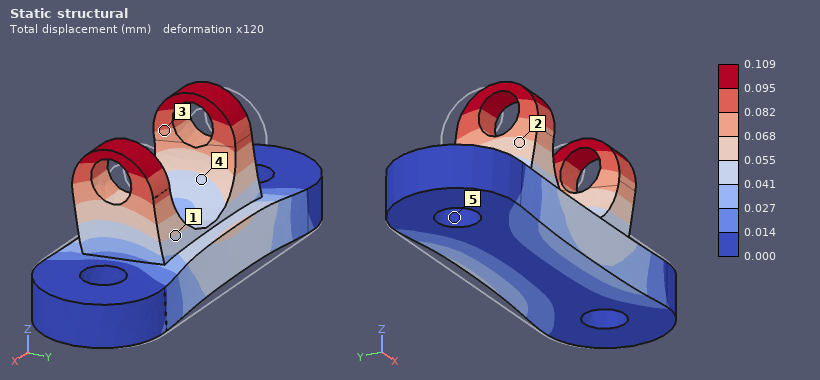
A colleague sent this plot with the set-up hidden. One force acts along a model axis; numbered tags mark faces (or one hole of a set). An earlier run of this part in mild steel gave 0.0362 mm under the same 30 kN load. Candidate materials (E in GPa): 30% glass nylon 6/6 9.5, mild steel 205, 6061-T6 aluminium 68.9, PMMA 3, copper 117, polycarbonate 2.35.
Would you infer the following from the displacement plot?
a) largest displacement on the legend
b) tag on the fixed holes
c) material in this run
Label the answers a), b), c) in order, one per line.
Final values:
a) 0.109 mm
b) 5
c) 6061-T6 aluminium
